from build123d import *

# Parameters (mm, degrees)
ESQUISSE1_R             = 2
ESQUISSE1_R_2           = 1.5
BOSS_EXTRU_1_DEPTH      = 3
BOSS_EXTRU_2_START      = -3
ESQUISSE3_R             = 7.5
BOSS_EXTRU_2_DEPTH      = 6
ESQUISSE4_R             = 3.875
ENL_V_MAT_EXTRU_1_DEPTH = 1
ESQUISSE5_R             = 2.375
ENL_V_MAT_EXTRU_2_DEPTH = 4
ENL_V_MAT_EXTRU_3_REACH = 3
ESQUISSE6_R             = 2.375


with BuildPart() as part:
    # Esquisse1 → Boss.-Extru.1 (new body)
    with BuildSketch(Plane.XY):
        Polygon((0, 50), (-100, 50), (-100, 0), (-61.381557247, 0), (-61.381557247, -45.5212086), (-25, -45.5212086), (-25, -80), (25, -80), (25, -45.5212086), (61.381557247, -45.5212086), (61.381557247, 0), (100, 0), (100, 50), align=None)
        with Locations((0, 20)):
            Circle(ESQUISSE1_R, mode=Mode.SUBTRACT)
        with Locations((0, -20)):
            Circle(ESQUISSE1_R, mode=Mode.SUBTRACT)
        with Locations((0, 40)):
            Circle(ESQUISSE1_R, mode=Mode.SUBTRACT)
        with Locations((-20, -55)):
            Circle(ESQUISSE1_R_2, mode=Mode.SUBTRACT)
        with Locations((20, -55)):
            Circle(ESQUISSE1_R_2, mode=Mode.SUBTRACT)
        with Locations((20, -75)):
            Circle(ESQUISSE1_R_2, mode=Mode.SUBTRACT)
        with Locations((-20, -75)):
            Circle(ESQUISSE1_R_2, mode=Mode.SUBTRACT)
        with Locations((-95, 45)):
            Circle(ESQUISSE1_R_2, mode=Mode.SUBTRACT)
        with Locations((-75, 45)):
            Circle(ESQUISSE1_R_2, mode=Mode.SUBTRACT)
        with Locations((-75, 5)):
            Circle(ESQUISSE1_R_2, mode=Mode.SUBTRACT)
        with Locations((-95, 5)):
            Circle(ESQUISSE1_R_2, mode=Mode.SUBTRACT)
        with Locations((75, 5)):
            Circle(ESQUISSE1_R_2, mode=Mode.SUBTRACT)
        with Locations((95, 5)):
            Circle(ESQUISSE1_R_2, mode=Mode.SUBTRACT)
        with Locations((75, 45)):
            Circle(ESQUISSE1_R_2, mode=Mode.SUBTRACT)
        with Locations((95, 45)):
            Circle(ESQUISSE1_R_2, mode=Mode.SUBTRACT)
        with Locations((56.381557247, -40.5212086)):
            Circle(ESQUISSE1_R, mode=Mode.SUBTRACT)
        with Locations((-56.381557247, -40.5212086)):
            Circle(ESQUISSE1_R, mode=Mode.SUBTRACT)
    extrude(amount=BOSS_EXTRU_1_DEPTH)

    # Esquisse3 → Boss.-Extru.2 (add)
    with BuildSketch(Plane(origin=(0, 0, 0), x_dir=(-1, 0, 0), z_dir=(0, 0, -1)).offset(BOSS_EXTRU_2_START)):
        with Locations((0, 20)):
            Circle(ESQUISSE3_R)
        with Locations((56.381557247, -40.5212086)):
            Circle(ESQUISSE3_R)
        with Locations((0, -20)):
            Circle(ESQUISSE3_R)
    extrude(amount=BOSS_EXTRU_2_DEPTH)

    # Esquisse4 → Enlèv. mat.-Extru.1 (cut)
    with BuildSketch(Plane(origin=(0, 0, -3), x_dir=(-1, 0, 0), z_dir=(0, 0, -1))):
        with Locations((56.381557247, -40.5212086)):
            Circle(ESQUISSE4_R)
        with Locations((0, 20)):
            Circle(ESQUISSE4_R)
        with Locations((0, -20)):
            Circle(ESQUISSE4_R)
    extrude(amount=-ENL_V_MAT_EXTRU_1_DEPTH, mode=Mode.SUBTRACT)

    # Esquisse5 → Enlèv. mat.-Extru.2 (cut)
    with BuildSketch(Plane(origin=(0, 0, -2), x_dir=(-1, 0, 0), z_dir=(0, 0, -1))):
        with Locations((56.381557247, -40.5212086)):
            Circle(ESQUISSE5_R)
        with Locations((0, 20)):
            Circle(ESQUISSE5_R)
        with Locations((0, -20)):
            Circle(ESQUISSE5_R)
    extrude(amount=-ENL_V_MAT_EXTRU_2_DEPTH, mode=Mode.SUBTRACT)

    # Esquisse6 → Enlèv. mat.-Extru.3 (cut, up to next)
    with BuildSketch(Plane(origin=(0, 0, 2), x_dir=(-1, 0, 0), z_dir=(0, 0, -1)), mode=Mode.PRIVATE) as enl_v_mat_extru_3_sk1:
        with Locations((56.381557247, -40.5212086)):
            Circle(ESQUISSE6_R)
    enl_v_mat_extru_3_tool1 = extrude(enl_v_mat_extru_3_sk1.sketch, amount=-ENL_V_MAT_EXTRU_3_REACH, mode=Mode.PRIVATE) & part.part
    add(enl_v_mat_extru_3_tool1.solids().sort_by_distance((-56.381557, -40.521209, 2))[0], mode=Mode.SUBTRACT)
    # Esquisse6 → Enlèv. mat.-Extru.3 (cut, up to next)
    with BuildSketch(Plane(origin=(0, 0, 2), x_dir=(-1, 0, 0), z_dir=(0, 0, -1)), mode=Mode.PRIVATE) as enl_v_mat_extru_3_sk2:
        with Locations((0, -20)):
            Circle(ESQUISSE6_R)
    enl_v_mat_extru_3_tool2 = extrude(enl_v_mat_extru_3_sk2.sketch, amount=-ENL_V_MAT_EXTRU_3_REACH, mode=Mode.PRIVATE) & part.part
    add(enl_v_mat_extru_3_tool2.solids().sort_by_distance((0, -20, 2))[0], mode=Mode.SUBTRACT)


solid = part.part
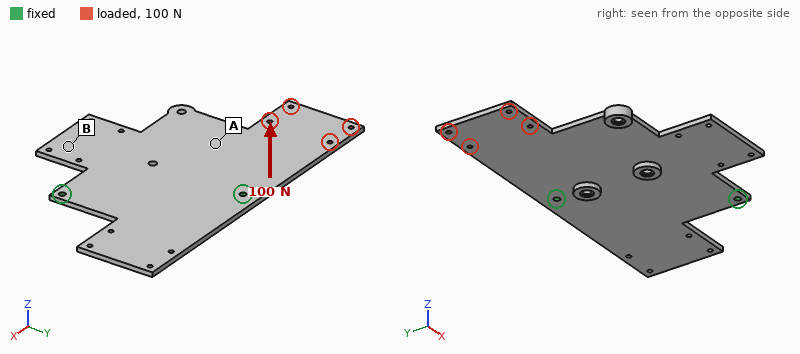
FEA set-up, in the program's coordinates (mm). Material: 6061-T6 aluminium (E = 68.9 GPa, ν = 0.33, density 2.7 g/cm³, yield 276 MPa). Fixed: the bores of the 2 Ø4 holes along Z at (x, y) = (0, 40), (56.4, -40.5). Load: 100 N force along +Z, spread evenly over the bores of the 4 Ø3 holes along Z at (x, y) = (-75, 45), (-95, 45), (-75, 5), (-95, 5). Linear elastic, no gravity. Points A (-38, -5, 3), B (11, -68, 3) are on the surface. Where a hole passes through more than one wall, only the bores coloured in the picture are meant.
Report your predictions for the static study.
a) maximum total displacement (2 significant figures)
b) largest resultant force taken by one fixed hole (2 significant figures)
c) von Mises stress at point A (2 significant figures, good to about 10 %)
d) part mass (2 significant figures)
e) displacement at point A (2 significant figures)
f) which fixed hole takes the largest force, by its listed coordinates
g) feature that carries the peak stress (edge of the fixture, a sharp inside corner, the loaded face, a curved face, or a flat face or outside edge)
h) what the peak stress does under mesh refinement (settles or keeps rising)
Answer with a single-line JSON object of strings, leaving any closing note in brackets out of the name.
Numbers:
{"maximum total displacement": "2.7 mm", "largest resultant force taken by one fixed hole": "140 N", "von Mises stress at point A": "33 MPa", "part mass": "140 g", "displacement at point A": "0.79 mm", "which fixed hole takes the largest force, by its listed coordinates": "(0, 40)", "feature that carries the peak stress": "edge of the fixture", "what the peak stress does under mesh refinement": "keeps rising"}
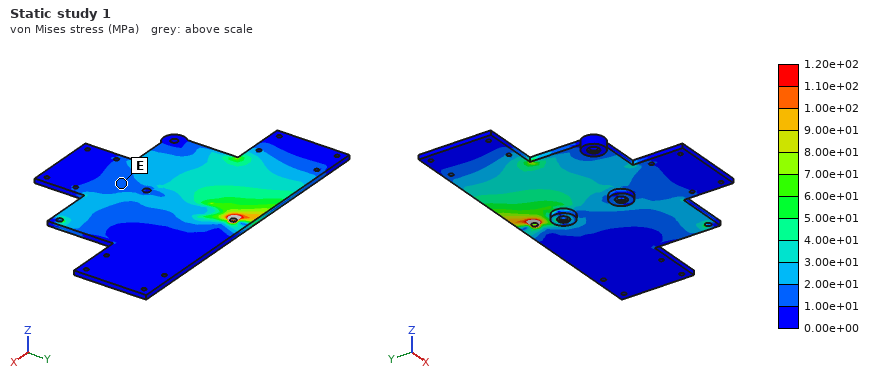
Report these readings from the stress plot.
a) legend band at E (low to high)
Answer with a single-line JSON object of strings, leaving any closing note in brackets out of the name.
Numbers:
{"legend band at E": "1.00e+01 to 2.00e+01 MPa"}
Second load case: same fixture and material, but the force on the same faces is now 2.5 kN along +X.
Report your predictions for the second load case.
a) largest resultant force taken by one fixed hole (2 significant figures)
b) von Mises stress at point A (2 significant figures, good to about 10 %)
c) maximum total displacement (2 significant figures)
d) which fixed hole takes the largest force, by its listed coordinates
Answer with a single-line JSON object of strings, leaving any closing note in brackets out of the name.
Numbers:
{"largest resultant force taken by one fixed hole": "1.9 kN", "von Mises stress at point A": "6.2 MPa", "maximum total displacement": "34 µm", "which fixed hole takes the largest force, by its listed coordinates": "(0, 40)"}
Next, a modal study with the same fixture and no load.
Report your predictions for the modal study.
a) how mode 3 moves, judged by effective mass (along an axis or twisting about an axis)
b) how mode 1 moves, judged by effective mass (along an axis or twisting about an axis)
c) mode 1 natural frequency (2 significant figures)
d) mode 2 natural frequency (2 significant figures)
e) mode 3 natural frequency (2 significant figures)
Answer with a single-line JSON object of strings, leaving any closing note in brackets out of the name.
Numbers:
{"how mode 3 moves, judged by effective mass": "along Z", "how mode 1 moves, judged by effective mass": "along Z", "mode 1 natural frequency": "210 Hz", "mode 2 natural frequency": "350 Hz", "mode 3 natural frequency": "410 Hz"}
